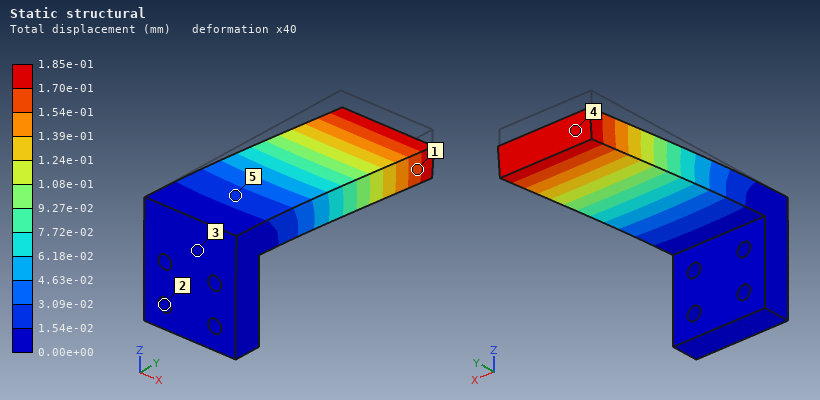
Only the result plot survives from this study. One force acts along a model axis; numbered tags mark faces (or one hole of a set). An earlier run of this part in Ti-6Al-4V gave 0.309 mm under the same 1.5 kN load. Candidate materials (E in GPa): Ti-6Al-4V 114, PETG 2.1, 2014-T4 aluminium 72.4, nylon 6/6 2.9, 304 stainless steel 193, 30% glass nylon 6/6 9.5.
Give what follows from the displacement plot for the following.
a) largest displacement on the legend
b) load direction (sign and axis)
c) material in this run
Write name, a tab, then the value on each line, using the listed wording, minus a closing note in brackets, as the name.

largest displacement on the legend	1.85e-01 mm
load direction	-Z
material in this run	304 stainless steel
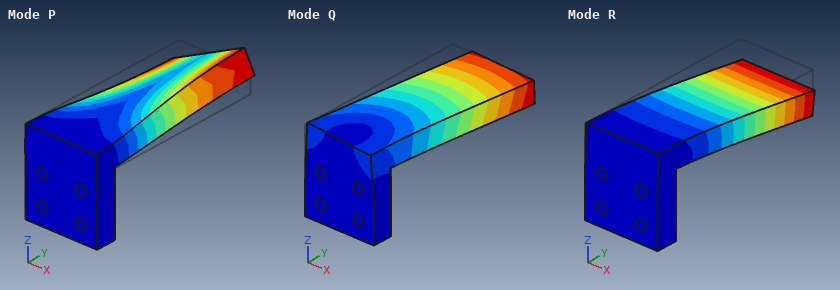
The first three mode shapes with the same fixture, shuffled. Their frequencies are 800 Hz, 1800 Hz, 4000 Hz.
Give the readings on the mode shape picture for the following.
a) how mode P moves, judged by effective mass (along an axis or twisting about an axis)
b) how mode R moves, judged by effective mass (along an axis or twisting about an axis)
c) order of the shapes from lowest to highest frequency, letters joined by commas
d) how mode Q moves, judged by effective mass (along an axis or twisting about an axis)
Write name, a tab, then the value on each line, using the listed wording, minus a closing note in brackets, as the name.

how mode P moves, judged by effective mass	twisting about Y
how mode R moves, judged by effective mass	along Z
order of the shapes from lowest to highest frequency, letters joined by commas	R, Q, P
how mode Q moves, judged by effective mass	along X
